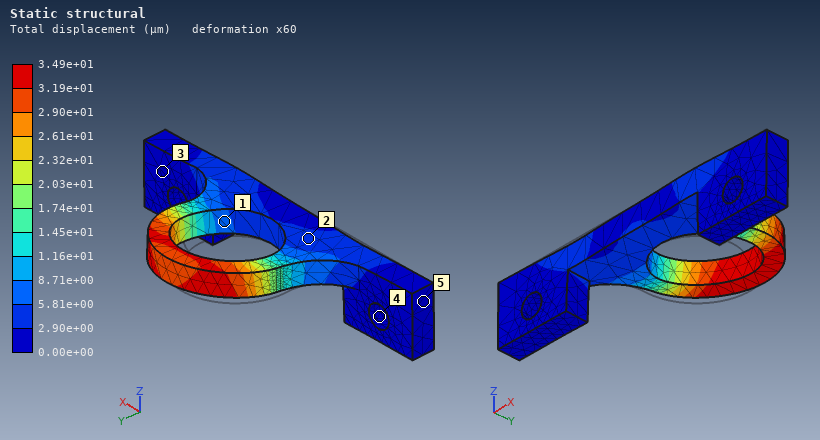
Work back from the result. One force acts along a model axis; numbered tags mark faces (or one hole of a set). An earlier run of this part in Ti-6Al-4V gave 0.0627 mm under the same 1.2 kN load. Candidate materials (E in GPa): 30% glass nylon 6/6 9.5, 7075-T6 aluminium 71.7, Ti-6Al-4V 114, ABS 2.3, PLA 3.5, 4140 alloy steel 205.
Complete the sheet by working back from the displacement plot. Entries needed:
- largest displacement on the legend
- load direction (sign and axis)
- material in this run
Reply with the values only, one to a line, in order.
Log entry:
3.49e+01 µm
+X
4140 alloy steel
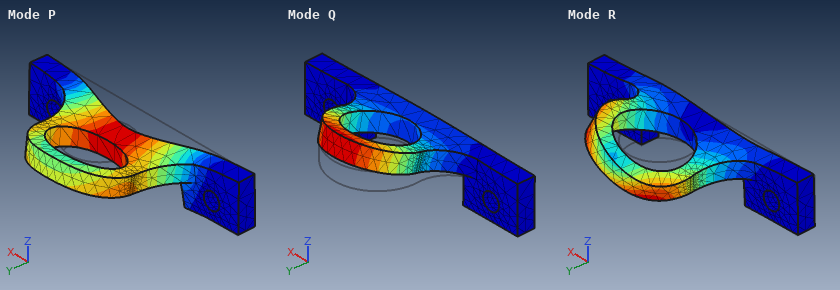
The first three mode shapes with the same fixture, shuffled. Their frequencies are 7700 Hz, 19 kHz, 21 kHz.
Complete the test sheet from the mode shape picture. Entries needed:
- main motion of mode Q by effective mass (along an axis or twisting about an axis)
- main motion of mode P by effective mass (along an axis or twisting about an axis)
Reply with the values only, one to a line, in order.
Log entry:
along Z
along Y
